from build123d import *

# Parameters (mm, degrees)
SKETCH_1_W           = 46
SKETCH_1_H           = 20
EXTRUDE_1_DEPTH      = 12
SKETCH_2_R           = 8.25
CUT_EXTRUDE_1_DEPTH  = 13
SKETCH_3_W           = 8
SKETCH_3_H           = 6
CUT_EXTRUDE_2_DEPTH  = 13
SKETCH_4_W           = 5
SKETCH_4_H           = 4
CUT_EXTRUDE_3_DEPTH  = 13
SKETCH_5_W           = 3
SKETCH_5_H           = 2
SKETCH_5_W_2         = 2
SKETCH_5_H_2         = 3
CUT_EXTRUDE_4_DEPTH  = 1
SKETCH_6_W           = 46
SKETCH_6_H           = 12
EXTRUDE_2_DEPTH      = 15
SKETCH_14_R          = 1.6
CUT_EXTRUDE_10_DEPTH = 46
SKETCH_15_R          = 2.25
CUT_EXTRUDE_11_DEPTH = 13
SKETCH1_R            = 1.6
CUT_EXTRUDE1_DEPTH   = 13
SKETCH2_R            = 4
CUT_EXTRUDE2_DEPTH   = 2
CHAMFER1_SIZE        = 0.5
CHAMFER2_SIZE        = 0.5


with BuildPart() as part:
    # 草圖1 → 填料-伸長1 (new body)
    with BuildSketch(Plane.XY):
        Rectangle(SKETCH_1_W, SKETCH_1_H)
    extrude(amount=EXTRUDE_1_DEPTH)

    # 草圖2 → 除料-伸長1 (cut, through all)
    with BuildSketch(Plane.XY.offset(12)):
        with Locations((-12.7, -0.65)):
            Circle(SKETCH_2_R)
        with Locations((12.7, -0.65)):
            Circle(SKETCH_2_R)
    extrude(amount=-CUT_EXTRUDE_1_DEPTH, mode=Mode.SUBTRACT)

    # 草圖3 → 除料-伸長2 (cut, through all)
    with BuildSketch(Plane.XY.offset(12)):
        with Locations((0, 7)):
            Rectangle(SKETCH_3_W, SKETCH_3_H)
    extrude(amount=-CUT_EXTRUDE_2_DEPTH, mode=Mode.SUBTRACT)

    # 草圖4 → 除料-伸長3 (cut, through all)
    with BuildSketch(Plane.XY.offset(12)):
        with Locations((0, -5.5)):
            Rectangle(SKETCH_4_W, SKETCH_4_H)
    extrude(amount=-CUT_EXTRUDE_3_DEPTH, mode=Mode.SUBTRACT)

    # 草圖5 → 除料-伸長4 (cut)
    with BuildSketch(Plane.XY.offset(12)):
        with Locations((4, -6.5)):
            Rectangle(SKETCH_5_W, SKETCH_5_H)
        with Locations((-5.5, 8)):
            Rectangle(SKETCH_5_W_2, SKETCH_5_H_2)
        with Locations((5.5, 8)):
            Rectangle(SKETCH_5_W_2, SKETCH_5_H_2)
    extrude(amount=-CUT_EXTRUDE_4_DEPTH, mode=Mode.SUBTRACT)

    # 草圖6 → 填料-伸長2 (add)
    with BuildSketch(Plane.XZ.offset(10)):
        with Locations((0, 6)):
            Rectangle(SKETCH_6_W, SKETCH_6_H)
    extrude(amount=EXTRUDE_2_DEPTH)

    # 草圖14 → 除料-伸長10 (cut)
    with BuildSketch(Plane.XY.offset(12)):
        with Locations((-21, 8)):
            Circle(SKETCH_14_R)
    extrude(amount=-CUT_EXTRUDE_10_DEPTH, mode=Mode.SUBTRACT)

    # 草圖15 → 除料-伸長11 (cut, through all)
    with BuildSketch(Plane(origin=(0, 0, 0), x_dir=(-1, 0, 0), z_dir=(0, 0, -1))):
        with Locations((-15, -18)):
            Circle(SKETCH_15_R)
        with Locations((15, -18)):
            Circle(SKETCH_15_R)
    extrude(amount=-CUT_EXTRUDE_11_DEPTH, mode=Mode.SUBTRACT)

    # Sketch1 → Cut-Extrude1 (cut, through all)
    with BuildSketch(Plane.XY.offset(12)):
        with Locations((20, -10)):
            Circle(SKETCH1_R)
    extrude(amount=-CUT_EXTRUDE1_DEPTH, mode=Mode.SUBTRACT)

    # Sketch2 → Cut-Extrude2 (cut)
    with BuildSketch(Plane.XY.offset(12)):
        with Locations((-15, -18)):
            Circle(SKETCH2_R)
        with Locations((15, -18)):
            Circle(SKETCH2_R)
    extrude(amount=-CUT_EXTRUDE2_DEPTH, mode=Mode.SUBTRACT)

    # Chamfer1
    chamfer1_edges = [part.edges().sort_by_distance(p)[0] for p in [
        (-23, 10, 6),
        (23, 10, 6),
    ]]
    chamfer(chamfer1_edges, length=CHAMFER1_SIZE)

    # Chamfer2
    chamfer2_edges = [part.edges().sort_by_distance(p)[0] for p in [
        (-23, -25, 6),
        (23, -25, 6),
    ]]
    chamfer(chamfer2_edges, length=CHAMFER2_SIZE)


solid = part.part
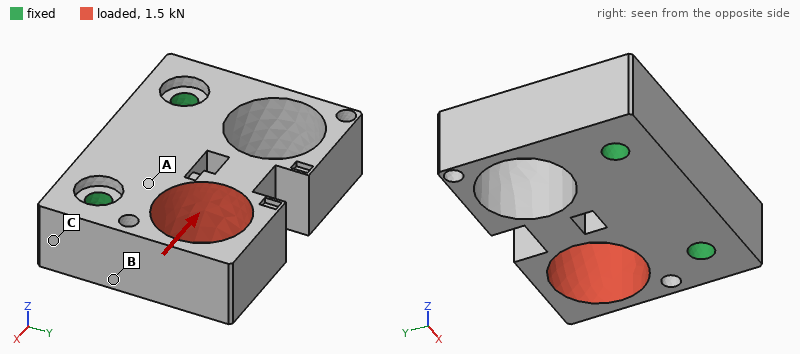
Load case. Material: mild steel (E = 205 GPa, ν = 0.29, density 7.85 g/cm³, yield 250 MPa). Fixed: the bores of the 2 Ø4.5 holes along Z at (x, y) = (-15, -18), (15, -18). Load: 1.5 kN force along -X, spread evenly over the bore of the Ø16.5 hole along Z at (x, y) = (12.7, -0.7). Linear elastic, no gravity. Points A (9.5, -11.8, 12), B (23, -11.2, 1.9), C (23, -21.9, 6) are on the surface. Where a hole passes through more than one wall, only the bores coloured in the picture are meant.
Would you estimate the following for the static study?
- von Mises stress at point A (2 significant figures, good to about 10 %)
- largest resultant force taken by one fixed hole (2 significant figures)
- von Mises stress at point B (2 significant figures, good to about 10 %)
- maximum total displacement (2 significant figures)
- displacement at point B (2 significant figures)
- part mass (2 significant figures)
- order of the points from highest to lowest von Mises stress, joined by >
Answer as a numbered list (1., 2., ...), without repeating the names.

1. 13 MPa
2. 1.1 kN
3. 27 MPa
4. 9.5 µm
5. 1.6 µm
6. 99 g
7. B > A > C
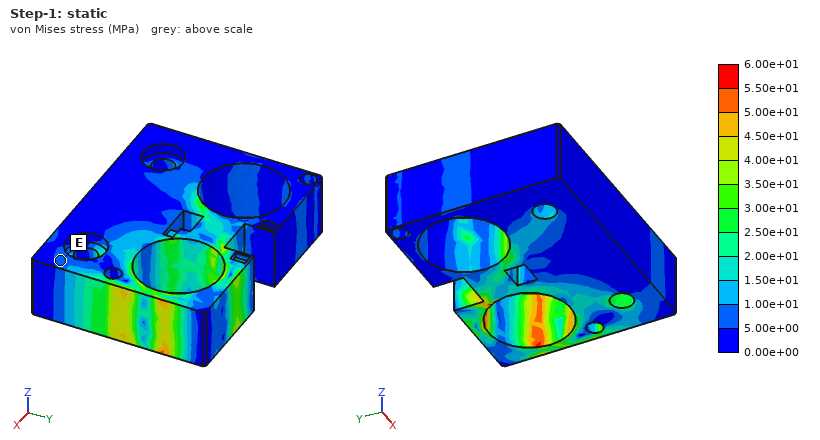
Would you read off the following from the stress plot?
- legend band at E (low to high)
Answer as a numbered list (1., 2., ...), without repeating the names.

1. 5.00e+00 to 1.00e+01 MPa
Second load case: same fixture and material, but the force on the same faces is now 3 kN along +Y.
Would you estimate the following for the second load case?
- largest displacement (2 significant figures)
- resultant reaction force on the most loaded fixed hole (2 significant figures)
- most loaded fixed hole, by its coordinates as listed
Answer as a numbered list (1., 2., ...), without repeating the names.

1. 11 µm
2. 2.6 kN
3. (15, -18)
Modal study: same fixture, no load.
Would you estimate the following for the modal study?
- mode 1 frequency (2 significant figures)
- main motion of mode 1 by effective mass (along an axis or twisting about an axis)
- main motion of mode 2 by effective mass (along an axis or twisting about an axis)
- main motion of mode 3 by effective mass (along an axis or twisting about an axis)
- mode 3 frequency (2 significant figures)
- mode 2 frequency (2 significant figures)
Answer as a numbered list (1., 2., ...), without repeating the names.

1. 9500 Hz
2. along Z
3. twisting about Y
4. along X
5. 14 kHz
6. 13 kHz
